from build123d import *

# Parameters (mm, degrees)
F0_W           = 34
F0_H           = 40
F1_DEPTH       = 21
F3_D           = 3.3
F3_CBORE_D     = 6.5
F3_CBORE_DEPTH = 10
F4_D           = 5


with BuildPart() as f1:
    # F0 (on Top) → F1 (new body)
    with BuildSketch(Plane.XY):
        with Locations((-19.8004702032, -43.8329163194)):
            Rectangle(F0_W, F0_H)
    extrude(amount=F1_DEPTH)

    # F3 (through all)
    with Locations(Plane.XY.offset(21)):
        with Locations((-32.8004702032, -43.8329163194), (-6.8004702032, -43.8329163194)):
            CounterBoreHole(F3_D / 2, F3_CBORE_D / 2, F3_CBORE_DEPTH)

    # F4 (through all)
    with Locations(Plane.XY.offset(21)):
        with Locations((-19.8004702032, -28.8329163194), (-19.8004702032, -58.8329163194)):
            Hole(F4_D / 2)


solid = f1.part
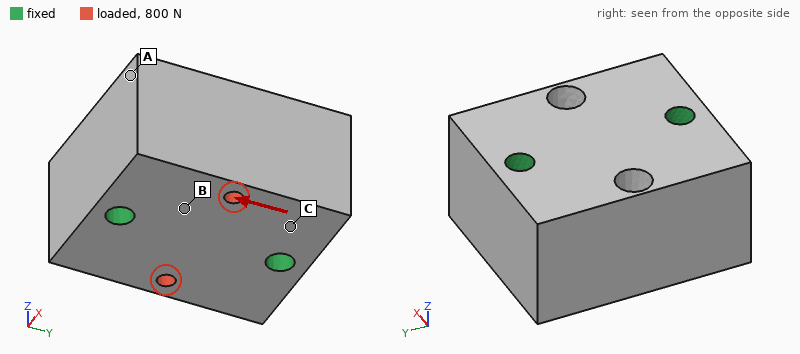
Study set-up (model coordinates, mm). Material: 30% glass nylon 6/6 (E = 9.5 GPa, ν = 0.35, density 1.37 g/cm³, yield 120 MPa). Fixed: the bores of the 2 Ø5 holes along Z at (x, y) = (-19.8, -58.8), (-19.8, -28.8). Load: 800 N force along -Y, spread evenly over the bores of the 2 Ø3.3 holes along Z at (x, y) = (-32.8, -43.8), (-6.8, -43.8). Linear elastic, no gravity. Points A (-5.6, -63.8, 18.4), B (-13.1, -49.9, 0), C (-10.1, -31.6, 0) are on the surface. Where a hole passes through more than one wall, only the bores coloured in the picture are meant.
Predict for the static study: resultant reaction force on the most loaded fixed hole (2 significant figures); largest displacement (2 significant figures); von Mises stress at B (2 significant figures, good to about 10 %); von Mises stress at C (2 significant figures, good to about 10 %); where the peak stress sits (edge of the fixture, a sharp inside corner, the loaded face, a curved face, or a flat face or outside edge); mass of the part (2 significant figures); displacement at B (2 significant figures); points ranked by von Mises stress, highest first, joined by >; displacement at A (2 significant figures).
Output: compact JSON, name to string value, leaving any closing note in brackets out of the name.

{"resultant reaction force on the most loaded fixed hole": "410 N", "largest displacement": "5.2 µm", "von Mises stress at B": "1.7 MPa", "von Mises stress at C": "1.2 MPa", "where the peak stress sits": "a sharp inside corner", "mass of the part": "37 g", "displacement at B": "1.8 µm", "points ranked by von Mises stress, highest first, joined by >": "B > C > A", "displacement at A": "2.0 µm"}
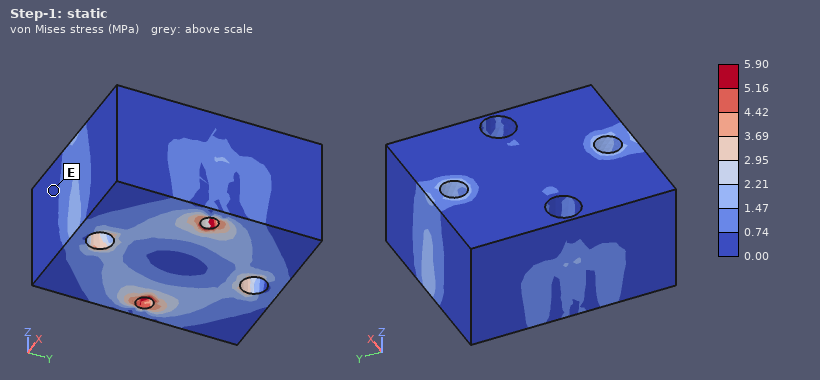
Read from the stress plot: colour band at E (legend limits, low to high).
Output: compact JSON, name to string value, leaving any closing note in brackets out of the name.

{"colour band at E": "0.00 to 0.74 MPa"}
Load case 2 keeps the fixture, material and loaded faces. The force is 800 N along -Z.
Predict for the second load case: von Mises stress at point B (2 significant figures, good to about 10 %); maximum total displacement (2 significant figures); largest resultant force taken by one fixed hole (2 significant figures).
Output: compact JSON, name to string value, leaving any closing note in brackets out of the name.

{"von Mises stress at point B": "1.9 MPa", "maximum total displacement": "10 µm", "largest resultant force taken by one fixed hole": "400 N"}
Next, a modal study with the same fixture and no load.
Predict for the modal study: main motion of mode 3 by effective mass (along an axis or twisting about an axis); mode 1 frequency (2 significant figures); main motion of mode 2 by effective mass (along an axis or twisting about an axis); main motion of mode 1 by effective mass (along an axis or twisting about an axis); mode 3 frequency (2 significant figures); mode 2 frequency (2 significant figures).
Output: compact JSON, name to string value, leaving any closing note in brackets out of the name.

{"main motion of mode 3 by effective mass": "along Y", "mode 1 frequency": "14 kHz", "main motion of mode 2 by effective mass": "along Z", "main motion of mode 1 by effective mass": "twisting about Y", "mode 3 frequency": "19 kHz", "mode 2 frequency": "16 kHz"}
